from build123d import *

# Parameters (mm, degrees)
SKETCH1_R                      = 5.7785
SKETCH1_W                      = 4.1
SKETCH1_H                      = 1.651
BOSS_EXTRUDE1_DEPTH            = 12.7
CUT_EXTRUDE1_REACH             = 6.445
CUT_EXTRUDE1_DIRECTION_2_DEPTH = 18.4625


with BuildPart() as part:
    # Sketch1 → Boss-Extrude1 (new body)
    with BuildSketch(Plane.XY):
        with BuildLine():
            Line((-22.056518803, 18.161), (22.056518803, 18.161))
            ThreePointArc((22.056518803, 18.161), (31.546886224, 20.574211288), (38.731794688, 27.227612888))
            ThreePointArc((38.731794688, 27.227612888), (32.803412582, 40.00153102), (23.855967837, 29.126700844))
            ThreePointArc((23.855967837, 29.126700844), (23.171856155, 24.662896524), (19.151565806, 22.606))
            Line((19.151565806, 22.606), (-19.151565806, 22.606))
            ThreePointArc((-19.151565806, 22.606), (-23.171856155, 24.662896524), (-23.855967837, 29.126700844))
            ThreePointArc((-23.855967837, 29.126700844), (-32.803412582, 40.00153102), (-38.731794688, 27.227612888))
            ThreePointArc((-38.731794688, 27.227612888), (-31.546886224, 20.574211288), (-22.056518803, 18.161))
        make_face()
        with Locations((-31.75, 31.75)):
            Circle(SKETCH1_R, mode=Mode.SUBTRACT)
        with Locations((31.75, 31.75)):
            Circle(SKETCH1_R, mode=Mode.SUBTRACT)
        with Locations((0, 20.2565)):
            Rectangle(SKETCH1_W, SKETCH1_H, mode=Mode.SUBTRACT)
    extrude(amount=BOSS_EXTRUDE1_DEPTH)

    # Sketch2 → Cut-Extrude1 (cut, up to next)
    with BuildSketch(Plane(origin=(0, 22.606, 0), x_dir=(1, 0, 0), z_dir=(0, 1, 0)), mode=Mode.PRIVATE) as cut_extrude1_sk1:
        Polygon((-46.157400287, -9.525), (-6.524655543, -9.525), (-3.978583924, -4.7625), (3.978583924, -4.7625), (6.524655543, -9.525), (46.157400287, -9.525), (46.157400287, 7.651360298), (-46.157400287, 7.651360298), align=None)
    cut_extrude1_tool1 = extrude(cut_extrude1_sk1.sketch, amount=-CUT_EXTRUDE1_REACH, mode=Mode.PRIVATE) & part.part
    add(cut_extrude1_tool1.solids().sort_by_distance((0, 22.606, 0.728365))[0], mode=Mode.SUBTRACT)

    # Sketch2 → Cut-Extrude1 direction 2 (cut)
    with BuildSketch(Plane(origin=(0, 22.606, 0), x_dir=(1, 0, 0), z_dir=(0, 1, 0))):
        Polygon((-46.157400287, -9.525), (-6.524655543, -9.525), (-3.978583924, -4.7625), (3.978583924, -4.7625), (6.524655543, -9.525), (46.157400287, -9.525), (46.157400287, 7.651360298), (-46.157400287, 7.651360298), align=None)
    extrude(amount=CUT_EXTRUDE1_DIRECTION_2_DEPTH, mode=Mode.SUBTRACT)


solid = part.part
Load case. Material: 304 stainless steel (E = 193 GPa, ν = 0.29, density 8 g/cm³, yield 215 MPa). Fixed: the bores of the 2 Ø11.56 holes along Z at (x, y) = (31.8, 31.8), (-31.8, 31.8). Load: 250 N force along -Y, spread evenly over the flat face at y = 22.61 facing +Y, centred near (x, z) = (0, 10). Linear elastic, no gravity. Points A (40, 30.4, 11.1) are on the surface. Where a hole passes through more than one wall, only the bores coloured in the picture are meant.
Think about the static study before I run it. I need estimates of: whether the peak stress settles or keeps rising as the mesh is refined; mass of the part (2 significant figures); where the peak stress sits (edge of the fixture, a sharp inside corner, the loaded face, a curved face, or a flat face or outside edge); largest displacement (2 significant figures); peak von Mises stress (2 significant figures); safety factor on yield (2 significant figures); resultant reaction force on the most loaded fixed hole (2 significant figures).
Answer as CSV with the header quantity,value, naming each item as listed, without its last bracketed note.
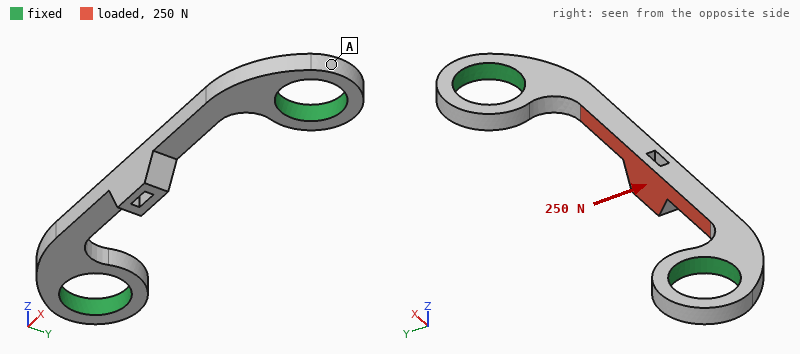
quantity,value
whether the peak stress settles or keeps rising as the mesh is refined,settles
mass of the part,15 g
where the peak stress sits,a curved face
largest displacement,32 µm
peak von Mises stress,100 MPa
safety factor on yield,2.1
resultant reaction force on the most loaded fixed hole,170 N
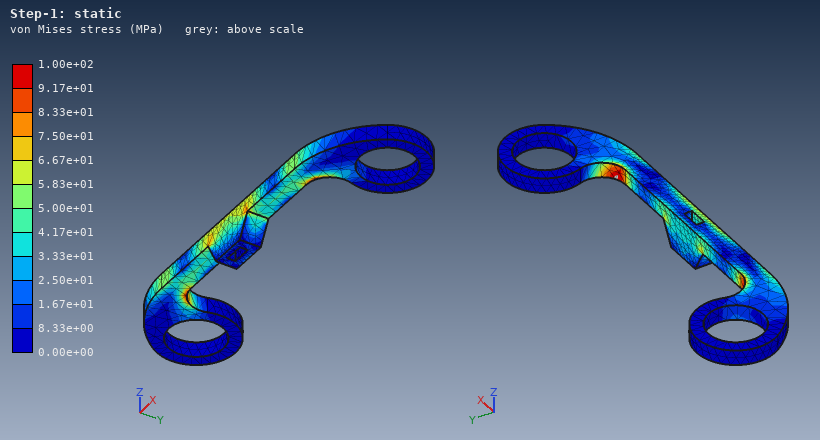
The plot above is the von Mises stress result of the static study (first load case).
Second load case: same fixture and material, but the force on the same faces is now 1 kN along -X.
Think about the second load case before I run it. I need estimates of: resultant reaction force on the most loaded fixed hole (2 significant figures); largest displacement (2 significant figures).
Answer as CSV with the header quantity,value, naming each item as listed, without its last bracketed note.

quantity,value
resultant reaction force on the most loaded fixed hole,500 N
largest displacement,13 µm
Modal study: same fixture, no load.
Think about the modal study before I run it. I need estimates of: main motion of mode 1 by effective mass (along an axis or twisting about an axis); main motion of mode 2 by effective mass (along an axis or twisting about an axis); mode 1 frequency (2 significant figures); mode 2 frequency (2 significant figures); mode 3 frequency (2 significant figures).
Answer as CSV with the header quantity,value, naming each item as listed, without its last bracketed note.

quantity,value
main motion of mode 1 by effective mass,along Z
main motion of mode 2 by effective mass,along Y
mode 1 frequency,4600 Hz
mode 2 frequency,7200 Hz
mode 3 frequency,12 kHz
